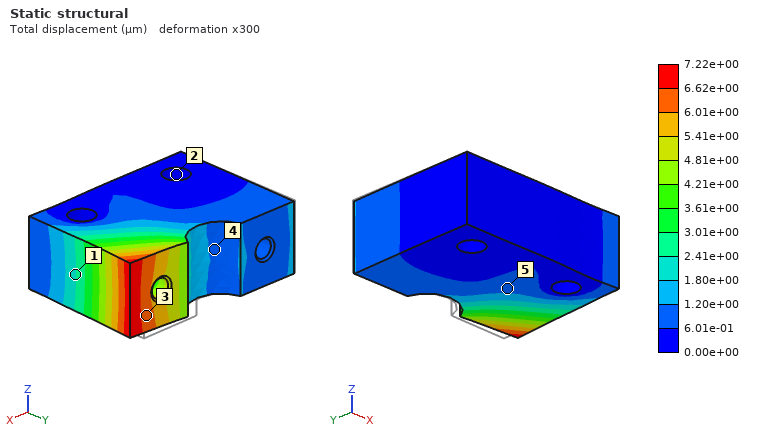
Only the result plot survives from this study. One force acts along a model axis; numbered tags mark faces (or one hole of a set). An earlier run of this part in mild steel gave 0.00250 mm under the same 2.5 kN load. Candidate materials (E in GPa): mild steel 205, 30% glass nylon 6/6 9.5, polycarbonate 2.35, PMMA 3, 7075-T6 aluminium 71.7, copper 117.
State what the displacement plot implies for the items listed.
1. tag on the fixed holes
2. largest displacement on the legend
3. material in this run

2
7.22e+00 µm
7075-T6 aluminium
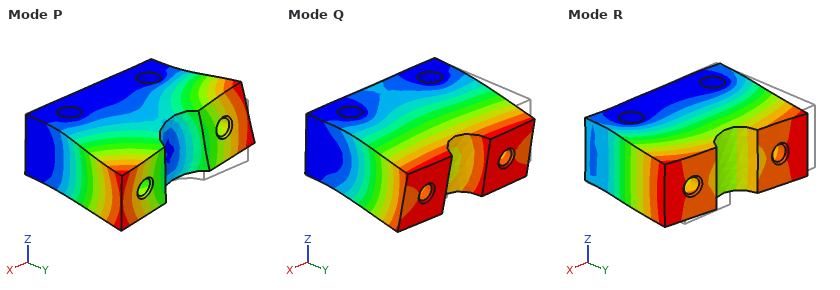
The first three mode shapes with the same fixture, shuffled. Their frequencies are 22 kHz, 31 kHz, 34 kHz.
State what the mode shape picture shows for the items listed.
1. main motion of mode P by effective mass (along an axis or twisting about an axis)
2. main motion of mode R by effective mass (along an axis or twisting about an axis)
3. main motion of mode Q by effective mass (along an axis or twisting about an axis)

twisting about Y
along X
along Z
